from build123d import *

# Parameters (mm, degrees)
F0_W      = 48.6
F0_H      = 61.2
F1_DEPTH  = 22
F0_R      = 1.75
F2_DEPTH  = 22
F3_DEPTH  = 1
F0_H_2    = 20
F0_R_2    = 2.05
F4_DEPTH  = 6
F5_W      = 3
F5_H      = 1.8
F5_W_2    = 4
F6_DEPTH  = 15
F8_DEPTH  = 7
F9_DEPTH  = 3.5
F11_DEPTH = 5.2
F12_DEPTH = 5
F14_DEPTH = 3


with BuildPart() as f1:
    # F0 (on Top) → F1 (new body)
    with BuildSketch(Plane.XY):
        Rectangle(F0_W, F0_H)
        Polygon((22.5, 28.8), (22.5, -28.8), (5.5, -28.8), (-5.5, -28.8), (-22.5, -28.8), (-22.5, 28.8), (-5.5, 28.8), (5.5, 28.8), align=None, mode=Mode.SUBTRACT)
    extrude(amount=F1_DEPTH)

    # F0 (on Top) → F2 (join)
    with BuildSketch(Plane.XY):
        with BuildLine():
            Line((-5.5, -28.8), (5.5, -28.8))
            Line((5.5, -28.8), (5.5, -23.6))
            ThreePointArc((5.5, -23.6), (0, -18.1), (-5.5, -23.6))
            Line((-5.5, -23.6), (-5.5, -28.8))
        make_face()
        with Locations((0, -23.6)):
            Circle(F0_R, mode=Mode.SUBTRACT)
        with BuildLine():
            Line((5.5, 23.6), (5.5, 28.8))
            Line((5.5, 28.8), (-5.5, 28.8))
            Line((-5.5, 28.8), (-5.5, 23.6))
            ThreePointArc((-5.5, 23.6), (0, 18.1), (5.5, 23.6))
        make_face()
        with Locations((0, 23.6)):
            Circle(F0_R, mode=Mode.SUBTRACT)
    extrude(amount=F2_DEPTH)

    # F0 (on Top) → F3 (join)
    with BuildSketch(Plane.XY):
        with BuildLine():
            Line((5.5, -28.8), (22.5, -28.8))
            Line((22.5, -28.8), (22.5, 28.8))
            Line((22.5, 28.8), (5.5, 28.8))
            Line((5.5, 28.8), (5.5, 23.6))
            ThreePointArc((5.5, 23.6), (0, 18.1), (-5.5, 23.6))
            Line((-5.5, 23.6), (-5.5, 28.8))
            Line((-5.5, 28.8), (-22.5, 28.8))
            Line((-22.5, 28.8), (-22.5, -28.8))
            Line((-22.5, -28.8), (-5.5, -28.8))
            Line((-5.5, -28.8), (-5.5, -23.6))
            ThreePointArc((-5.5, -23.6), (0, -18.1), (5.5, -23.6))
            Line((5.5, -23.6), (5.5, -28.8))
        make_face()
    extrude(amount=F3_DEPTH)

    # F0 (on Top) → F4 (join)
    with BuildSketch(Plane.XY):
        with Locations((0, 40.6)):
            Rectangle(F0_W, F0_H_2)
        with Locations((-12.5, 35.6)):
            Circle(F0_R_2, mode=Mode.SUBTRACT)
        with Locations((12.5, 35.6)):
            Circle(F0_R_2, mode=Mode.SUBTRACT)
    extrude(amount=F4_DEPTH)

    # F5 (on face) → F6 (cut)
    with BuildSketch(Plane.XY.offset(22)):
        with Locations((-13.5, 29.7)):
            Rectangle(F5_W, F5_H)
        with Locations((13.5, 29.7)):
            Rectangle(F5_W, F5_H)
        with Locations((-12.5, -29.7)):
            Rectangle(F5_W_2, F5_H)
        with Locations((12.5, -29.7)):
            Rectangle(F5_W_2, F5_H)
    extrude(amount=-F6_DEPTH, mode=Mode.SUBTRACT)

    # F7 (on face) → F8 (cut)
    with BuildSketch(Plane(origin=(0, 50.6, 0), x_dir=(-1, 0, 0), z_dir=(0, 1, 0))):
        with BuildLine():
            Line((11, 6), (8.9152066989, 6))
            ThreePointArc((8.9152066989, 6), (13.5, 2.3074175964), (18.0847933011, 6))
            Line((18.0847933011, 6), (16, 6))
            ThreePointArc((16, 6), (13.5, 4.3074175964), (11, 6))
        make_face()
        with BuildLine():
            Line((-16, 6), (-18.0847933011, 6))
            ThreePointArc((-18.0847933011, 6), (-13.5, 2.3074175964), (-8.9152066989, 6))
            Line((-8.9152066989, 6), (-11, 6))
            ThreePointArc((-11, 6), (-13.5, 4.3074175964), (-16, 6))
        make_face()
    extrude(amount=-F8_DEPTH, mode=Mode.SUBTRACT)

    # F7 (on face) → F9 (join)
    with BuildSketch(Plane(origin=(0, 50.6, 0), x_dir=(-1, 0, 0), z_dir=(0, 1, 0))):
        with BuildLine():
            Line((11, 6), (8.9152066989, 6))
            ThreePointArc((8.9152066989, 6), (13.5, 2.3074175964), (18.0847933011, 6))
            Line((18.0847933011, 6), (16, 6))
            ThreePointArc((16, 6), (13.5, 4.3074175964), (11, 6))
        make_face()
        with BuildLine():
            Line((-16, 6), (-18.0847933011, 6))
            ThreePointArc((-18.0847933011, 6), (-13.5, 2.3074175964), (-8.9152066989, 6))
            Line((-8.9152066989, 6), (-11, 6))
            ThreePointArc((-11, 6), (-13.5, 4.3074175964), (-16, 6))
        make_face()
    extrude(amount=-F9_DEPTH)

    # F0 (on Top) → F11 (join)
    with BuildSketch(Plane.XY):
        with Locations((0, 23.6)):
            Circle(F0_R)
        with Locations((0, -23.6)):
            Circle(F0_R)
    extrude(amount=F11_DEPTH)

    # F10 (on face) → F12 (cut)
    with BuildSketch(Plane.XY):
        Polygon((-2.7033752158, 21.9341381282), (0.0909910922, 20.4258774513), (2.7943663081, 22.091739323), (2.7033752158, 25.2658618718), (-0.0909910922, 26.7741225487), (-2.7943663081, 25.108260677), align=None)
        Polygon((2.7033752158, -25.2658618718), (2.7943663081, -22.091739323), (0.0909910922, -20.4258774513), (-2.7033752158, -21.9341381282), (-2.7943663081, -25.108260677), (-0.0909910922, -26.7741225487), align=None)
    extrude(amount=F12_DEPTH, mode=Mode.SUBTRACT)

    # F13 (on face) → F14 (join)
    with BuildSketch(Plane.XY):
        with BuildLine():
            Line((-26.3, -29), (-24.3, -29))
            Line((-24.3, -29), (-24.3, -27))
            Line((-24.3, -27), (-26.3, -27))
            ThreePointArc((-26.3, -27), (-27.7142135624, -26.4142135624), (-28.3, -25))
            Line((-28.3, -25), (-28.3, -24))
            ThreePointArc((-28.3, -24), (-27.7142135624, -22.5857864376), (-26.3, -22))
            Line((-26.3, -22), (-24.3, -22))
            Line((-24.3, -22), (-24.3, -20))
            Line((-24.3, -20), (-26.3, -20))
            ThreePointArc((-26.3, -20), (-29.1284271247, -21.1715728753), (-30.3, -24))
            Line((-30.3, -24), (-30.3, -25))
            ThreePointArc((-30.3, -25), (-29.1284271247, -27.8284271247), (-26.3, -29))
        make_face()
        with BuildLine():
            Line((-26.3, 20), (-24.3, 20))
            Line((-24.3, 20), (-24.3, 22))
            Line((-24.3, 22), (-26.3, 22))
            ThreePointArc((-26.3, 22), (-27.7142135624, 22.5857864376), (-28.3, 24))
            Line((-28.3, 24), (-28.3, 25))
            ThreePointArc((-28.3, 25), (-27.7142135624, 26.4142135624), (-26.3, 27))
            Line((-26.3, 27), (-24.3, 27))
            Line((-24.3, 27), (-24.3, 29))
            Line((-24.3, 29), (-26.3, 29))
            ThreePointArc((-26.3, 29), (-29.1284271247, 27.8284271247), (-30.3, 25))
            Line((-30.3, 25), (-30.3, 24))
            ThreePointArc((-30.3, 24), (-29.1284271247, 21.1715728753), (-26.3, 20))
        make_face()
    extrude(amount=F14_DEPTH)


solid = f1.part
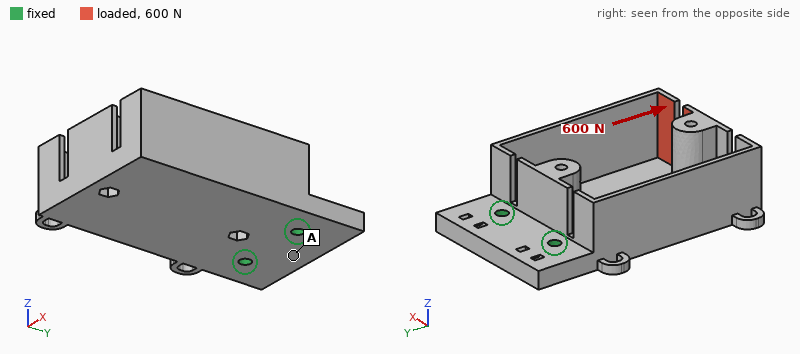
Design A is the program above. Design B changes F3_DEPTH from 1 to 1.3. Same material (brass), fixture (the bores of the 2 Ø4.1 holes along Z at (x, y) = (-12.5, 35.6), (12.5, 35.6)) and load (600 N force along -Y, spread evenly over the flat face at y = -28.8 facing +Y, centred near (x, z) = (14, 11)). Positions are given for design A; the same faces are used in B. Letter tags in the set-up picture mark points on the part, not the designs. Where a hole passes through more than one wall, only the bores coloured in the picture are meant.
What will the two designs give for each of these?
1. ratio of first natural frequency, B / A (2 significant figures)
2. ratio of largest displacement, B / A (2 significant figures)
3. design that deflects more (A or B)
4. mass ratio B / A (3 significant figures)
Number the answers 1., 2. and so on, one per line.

1. 1.0
2. 0.82
3. A
4. 1.04
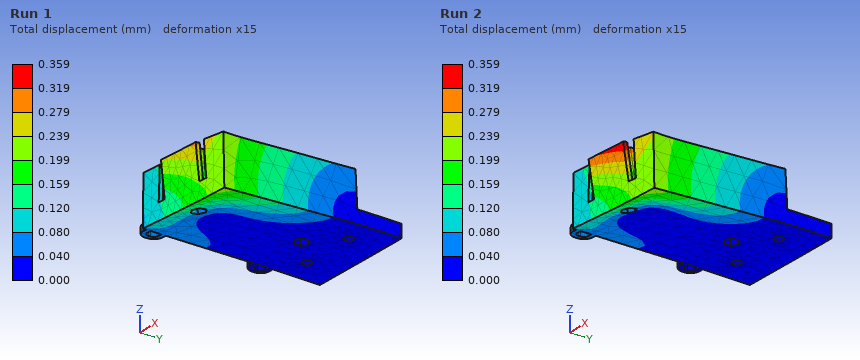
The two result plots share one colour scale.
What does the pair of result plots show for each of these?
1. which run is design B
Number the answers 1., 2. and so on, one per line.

1. Run 1
